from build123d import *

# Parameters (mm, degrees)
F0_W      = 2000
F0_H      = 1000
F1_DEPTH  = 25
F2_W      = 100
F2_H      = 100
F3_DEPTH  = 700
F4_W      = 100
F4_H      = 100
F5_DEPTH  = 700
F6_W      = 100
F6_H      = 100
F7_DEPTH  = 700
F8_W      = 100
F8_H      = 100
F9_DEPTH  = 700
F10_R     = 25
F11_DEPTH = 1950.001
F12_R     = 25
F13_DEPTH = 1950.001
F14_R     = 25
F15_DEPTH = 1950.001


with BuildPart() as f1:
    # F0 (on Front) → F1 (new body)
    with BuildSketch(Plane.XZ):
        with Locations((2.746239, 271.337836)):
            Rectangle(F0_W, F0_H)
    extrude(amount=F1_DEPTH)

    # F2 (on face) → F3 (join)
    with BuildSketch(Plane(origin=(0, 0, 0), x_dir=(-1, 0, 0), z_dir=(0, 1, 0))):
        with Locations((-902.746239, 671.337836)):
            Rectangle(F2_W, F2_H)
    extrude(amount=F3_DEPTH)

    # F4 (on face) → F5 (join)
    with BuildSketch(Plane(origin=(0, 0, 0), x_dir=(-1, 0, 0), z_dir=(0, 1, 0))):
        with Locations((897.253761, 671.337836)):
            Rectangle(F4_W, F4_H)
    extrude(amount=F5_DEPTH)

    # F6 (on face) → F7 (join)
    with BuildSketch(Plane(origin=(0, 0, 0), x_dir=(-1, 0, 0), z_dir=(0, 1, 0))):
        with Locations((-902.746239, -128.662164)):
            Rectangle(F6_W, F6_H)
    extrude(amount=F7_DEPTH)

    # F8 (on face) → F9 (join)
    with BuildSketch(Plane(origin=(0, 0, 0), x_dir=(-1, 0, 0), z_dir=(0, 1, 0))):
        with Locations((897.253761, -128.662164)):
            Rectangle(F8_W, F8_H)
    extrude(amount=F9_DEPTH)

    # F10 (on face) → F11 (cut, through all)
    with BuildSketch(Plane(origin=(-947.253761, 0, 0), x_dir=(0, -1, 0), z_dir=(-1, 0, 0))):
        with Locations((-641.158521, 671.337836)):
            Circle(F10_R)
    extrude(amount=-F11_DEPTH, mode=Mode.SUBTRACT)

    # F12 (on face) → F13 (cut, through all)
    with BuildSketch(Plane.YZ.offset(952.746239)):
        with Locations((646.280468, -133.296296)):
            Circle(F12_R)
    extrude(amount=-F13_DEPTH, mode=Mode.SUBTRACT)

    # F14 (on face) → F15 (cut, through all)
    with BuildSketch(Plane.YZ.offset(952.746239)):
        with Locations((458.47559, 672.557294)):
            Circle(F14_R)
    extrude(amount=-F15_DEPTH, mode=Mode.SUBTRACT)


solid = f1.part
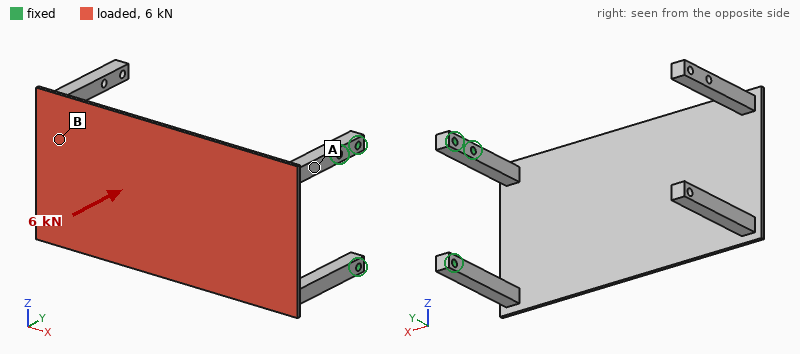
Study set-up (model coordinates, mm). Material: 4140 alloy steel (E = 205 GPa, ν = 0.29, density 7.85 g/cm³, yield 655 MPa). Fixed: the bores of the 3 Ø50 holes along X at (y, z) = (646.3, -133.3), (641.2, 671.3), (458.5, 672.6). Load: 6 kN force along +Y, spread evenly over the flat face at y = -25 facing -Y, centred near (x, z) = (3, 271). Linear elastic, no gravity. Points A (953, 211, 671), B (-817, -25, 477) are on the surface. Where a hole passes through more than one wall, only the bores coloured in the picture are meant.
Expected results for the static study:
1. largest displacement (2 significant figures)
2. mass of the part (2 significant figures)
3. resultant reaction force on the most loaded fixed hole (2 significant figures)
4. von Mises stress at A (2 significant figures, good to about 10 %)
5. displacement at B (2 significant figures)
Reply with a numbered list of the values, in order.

1. 22 mm
2. 600 kg
3. 3.5 kN
4. 17 MPa
5. 18 mm
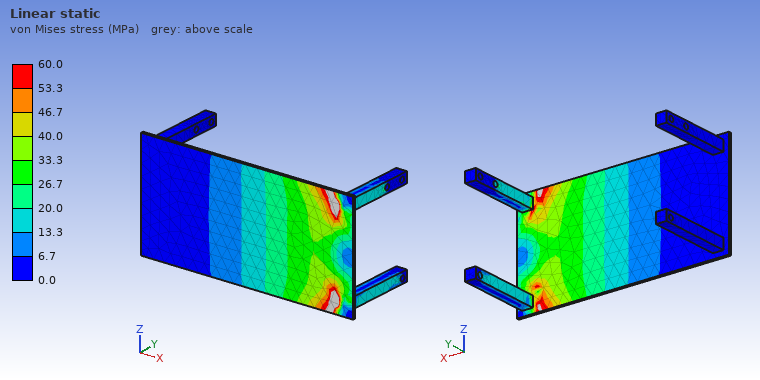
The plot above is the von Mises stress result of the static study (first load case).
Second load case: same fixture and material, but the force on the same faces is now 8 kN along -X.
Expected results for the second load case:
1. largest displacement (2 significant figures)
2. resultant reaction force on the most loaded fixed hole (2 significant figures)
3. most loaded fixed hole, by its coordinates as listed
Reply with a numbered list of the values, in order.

1. 1.2 mm
2. 5.2 kN
3. (458.5, 672.6)
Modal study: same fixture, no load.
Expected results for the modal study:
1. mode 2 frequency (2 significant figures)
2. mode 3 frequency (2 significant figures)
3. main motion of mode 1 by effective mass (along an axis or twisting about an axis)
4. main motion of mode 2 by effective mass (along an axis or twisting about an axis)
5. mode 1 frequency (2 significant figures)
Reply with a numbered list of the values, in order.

1. 12 Hz
2. 20 Hz
3. along Y
4. along Z
5. 3.8 Hz
